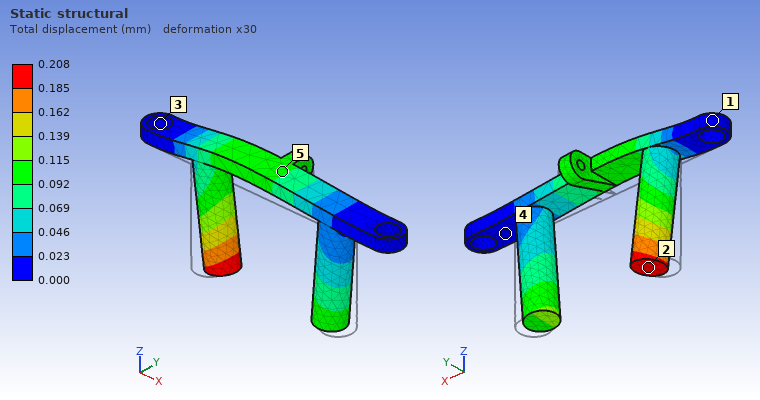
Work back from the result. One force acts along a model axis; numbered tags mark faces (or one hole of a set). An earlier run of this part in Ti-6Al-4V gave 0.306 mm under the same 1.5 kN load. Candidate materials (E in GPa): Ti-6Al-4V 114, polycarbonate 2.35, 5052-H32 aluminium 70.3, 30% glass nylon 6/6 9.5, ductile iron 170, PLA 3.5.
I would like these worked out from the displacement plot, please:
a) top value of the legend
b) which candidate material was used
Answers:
0.208 mm
ductile iron
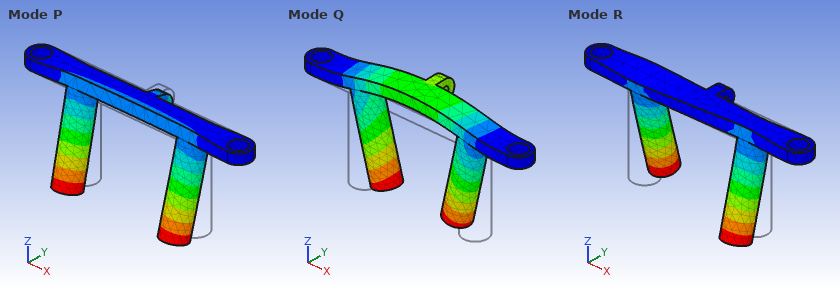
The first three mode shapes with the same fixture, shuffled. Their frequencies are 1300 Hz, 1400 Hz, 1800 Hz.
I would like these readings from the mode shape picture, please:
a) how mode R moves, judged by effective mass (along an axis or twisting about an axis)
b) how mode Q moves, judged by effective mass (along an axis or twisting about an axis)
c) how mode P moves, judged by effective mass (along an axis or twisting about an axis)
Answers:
twisting about Z
along Z
along Y
